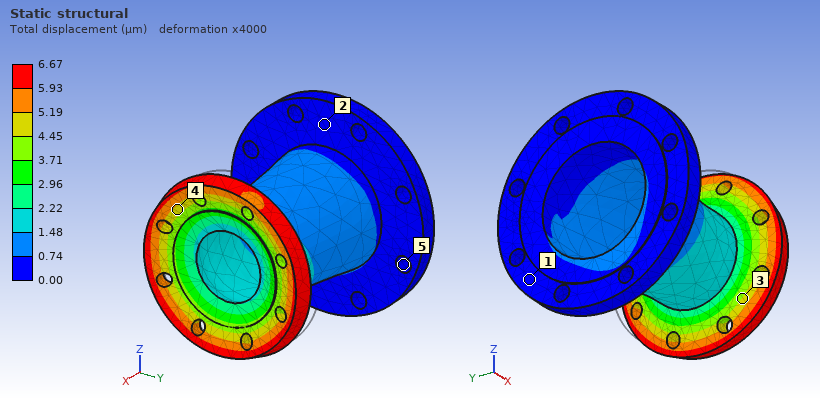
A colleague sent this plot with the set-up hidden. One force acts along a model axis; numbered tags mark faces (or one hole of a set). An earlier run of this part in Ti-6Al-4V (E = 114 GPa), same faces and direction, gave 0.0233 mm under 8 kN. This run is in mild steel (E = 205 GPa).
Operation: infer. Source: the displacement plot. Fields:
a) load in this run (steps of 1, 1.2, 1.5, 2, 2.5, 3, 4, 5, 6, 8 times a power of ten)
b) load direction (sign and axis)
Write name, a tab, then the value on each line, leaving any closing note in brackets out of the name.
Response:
load in this run	4 kN
load direction	+X
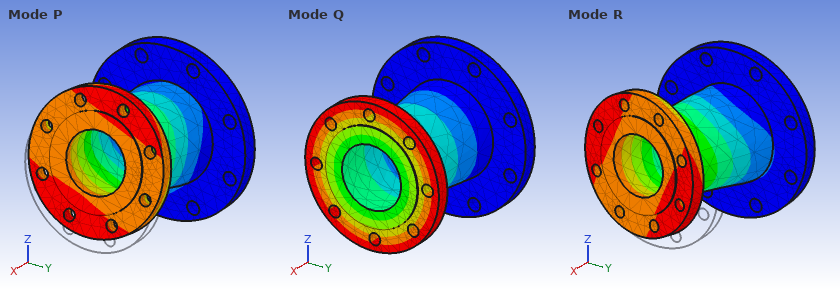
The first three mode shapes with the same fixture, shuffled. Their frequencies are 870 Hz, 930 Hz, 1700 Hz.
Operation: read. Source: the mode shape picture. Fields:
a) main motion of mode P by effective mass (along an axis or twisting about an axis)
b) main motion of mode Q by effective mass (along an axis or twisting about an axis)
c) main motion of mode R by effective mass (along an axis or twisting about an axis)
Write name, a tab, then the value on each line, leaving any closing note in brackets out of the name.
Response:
main motion of mode P by effective mass	along Z
main motion of mode Q by effective mass	twisting about X
main motion of mode R by effective mass	along Y
